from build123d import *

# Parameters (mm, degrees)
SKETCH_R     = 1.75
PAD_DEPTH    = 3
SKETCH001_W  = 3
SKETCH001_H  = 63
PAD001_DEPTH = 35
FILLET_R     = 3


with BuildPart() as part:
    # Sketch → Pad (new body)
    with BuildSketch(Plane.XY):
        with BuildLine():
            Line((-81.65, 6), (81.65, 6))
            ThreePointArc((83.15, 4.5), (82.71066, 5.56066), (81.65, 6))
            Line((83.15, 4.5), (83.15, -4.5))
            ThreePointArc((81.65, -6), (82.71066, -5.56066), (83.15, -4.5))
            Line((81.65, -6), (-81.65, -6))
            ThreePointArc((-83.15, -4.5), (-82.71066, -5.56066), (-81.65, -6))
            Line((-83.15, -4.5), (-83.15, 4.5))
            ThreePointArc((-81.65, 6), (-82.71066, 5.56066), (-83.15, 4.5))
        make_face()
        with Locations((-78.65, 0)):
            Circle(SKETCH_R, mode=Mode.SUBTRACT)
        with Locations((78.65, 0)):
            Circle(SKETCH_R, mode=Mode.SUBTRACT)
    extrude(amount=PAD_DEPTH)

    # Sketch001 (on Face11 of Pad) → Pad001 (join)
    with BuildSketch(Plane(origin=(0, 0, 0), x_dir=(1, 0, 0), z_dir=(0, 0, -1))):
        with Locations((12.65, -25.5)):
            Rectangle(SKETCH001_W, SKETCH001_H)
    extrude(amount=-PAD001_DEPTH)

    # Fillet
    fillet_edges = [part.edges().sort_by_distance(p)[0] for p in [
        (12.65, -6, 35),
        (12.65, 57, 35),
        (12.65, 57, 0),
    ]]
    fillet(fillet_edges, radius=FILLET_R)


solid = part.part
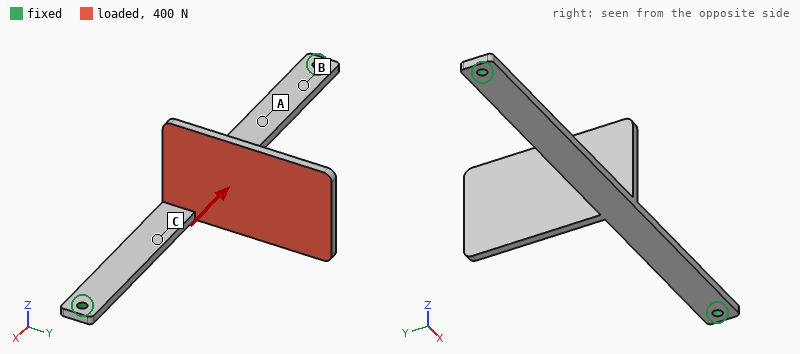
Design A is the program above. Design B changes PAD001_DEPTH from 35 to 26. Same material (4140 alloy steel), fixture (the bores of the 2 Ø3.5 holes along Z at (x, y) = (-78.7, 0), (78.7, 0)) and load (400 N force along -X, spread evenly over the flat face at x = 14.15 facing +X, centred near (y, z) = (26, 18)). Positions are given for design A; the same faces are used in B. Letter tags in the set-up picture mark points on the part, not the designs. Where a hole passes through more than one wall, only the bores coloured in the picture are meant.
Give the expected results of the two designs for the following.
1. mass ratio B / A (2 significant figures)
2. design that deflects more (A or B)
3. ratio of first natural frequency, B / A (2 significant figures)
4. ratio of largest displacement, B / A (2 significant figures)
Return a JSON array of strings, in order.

["0.86", "A", "1.2", "0.83"]
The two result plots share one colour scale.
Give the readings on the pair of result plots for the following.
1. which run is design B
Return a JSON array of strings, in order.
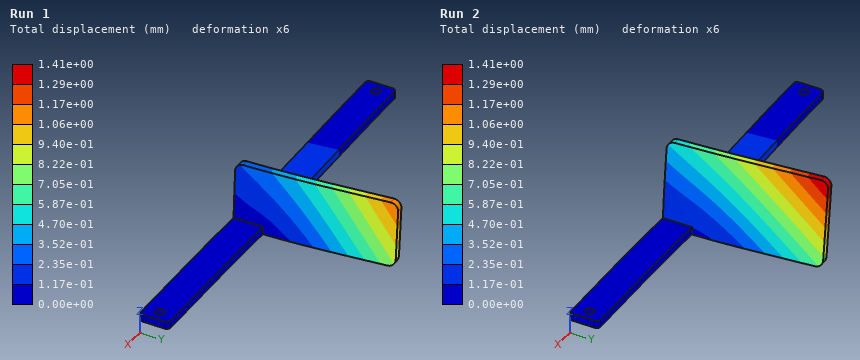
["Run 1"]
